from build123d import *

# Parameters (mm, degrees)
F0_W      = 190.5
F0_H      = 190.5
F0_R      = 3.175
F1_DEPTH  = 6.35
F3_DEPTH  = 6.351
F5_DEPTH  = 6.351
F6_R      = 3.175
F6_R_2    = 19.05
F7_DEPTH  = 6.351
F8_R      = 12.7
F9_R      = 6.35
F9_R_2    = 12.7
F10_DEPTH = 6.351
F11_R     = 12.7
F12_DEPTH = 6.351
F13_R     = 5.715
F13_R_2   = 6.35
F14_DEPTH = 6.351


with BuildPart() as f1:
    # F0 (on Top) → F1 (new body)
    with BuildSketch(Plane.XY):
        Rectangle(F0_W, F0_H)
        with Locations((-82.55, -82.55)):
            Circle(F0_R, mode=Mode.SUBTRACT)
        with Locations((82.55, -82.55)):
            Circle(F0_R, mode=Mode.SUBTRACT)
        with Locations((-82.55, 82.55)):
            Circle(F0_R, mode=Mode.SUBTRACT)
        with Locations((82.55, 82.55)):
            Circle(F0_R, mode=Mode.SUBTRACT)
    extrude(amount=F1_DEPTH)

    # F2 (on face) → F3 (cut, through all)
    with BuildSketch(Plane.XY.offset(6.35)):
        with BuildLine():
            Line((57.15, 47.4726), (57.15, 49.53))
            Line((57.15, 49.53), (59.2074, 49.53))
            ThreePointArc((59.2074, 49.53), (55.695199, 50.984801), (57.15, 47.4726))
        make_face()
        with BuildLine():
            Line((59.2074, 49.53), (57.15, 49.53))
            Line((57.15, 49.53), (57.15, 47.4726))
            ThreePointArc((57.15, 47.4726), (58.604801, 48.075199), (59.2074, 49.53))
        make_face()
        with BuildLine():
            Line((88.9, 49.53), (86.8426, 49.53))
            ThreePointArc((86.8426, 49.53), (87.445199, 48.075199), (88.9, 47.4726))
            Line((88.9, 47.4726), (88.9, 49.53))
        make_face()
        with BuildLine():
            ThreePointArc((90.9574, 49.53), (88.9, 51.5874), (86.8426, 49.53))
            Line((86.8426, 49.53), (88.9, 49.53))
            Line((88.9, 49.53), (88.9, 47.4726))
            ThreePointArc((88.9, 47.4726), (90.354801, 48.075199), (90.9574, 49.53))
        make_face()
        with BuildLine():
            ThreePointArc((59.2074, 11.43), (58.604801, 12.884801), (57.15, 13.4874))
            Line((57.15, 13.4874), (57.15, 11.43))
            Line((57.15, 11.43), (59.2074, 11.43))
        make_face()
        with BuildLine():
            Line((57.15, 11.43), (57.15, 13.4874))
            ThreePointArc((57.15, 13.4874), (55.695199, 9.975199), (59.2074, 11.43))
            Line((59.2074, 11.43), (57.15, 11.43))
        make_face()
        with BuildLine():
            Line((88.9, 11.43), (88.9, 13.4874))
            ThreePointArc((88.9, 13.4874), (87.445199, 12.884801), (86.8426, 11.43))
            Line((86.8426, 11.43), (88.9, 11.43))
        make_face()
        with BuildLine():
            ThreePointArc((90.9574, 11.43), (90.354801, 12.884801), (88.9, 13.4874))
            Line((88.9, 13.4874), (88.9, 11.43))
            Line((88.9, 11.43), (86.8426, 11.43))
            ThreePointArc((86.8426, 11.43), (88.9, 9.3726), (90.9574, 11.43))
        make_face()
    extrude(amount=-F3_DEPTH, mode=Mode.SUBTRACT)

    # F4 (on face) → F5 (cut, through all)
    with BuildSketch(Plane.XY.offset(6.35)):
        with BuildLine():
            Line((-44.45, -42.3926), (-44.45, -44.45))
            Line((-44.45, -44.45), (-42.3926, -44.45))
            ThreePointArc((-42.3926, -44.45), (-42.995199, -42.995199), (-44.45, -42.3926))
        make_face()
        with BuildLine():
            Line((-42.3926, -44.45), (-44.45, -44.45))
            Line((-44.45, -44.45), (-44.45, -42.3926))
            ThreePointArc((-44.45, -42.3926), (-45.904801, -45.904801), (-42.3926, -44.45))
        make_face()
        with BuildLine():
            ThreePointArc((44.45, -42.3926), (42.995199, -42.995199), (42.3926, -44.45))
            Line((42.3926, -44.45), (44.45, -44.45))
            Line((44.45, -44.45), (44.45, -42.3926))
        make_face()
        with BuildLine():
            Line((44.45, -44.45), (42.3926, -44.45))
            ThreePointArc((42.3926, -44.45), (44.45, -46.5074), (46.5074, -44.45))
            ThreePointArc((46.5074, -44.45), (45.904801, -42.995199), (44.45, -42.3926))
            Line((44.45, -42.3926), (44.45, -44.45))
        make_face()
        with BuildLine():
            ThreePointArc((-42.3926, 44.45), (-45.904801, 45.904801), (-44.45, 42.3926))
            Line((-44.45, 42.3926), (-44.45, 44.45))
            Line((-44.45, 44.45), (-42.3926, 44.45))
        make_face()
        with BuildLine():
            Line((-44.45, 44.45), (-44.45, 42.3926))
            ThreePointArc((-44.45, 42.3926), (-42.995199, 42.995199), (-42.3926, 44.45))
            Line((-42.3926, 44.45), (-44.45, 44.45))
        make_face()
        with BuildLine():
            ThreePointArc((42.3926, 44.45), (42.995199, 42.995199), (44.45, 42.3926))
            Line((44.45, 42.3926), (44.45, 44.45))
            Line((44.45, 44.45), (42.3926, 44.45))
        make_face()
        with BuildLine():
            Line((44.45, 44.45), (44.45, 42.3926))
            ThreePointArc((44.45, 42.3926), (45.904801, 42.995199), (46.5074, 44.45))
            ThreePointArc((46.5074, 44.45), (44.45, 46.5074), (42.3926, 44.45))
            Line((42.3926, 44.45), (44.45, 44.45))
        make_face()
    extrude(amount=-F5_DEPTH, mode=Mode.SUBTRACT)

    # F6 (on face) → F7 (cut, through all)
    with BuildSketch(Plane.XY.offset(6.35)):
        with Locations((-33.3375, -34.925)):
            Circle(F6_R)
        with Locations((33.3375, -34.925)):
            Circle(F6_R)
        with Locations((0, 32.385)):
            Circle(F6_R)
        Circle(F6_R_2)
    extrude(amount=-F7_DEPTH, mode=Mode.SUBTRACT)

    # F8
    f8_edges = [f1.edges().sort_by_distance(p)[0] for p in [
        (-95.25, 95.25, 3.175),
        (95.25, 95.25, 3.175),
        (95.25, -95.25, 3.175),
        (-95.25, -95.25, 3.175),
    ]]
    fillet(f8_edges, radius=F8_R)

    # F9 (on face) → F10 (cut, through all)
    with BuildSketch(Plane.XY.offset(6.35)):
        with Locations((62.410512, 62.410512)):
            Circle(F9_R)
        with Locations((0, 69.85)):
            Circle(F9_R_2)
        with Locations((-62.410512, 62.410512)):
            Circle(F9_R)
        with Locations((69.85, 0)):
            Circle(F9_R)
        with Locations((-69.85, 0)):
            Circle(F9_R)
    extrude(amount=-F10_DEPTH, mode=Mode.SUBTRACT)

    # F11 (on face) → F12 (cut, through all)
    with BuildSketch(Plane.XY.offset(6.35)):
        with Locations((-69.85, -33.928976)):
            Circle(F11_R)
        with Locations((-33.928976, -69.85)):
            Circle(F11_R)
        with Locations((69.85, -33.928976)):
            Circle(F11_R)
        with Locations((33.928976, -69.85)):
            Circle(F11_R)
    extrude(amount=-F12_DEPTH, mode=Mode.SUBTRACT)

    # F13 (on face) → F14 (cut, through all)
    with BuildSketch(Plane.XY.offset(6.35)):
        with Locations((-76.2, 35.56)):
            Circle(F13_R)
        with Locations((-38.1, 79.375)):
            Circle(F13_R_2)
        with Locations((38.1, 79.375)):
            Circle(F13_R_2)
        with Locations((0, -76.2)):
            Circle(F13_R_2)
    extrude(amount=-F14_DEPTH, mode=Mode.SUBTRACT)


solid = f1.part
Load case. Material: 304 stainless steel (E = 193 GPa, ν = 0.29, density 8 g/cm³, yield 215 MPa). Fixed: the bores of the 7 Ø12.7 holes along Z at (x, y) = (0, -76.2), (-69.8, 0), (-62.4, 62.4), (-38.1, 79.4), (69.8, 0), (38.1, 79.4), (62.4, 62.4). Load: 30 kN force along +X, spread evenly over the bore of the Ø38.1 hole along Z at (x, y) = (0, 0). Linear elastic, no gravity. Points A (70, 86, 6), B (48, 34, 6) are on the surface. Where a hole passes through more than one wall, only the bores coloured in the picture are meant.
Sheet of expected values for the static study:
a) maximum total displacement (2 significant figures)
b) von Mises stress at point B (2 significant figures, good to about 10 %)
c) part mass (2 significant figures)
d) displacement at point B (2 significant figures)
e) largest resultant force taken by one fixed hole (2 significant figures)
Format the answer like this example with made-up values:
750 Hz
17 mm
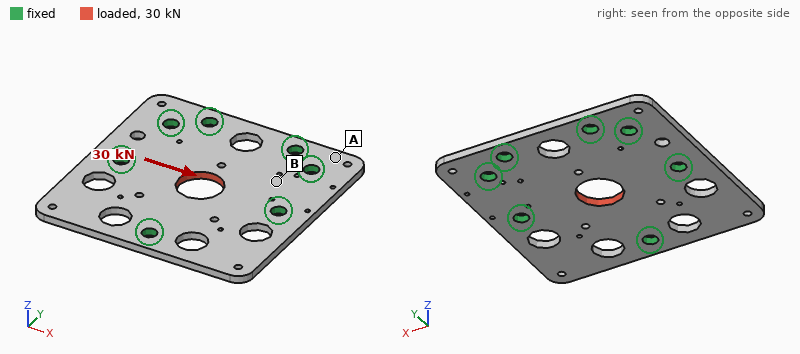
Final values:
13 µm
13 MPa
1.6 kg
3.1 µm
9.5 kN
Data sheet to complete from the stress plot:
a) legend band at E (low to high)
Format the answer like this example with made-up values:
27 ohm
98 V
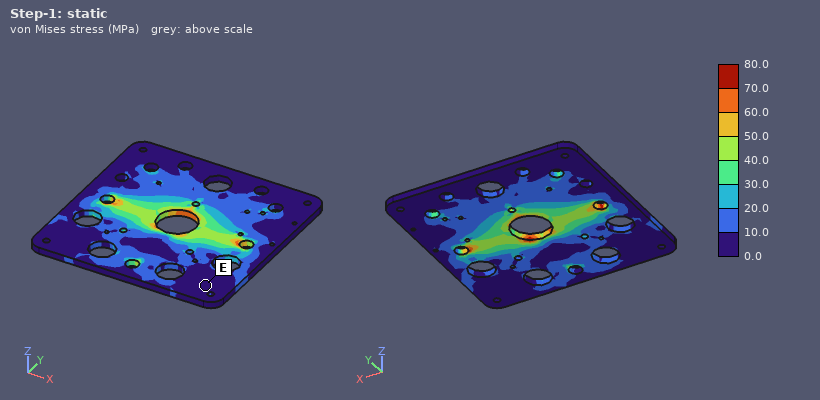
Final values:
0.0 to 10.0 MPa
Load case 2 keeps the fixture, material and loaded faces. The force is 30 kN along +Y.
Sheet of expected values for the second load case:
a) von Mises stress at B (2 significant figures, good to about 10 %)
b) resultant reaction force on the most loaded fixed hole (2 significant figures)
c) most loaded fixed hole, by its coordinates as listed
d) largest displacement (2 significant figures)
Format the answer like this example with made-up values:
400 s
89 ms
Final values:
19 MPa
8.7 kN
(0, -76.2)
12 µm
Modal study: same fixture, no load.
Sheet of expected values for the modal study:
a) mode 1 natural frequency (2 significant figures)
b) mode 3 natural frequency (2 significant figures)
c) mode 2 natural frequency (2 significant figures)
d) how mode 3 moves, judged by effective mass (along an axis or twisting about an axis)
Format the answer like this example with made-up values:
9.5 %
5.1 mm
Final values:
1100 Hz
2400 Hz
1100 Hz
along Z
